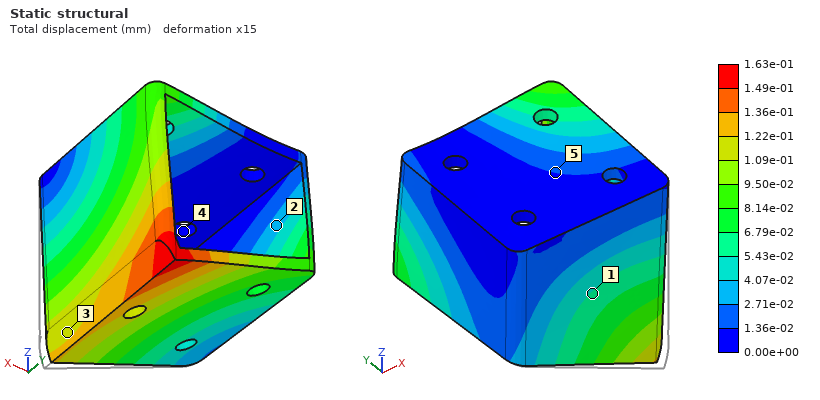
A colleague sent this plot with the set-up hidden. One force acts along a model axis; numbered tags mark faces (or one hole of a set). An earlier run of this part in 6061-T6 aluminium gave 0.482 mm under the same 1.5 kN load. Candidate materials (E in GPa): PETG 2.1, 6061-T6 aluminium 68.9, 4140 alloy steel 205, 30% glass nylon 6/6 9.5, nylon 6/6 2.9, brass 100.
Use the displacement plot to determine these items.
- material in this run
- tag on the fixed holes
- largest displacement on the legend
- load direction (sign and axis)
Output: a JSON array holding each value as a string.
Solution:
["4140 alloy steel", "4", "1.63e-01 mm", "+Y"]
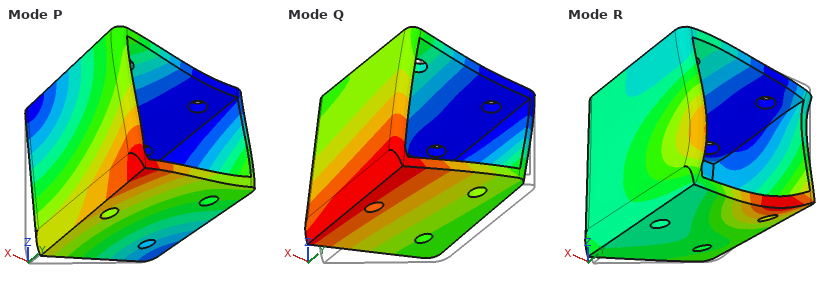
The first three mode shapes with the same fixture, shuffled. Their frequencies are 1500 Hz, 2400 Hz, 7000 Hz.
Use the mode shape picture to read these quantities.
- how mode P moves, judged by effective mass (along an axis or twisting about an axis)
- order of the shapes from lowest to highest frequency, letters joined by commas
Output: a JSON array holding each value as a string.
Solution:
["along Y", "Q, P, R"]
